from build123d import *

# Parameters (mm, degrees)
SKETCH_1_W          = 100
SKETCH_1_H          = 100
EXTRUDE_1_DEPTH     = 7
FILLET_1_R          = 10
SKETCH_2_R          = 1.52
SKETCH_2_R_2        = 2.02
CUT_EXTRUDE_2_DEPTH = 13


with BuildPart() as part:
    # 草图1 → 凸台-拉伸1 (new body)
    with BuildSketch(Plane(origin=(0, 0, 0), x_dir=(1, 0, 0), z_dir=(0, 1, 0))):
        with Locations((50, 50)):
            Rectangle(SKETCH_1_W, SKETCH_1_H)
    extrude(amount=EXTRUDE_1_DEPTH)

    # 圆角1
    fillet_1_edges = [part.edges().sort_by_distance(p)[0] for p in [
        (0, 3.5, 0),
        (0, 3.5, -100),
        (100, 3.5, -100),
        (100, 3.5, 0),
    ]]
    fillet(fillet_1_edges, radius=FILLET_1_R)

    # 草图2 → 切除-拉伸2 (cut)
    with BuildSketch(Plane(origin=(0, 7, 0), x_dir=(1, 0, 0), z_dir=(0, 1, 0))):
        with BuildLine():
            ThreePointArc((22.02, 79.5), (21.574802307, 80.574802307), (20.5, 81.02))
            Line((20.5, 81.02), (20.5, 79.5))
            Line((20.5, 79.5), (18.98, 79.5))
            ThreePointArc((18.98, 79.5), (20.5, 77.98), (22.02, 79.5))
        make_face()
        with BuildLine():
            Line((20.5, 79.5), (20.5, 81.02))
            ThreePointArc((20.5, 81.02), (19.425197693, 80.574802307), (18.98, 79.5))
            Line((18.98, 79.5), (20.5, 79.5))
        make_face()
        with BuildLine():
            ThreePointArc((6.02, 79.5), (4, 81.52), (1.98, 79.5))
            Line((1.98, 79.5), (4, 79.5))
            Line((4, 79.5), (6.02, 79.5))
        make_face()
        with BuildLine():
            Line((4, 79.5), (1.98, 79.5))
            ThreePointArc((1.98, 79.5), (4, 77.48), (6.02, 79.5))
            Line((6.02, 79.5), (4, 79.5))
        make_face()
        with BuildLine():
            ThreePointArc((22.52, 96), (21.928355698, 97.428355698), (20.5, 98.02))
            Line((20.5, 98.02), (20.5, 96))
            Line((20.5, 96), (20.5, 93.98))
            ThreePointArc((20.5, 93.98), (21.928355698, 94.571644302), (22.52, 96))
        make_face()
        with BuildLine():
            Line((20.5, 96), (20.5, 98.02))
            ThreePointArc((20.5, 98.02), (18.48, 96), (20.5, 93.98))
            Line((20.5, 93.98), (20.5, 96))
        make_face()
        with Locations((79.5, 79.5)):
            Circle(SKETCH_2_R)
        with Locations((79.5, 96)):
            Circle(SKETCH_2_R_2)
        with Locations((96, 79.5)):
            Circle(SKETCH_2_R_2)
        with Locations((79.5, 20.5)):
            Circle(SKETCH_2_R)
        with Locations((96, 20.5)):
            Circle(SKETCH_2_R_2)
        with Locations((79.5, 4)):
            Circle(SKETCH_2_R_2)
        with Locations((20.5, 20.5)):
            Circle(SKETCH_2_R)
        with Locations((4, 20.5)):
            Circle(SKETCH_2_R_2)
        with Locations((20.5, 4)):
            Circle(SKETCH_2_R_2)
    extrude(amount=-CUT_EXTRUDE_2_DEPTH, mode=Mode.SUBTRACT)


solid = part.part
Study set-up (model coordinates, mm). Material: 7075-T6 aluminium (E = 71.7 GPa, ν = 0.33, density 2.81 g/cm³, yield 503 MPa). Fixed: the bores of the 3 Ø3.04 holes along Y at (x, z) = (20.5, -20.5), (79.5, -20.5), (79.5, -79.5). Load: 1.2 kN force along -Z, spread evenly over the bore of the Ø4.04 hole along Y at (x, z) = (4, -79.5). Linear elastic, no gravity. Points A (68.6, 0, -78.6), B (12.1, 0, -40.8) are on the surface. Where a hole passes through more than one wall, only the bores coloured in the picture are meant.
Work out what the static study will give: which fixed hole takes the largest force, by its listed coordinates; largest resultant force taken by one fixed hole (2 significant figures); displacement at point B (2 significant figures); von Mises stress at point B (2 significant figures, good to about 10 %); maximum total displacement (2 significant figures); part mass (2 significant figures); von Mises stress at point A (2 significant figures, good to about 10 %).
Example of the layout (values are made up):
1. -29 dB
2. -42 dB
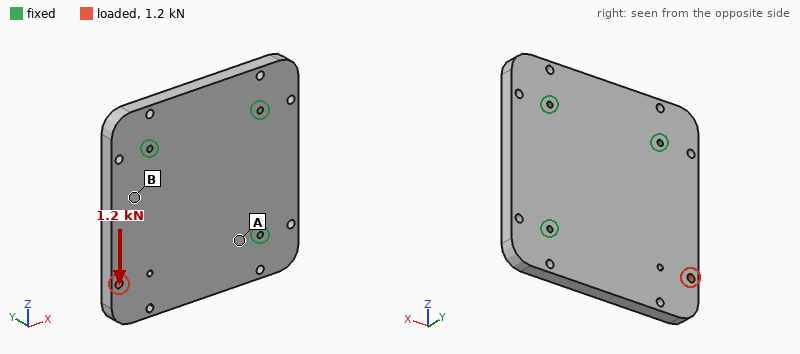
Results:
1. (20.5, -20.5)
2. 1.1 kN
3. 2.6 µm
4. 5.9 MPa
5. 8.9 µm
6. 190 g
7. 2.7 MPa
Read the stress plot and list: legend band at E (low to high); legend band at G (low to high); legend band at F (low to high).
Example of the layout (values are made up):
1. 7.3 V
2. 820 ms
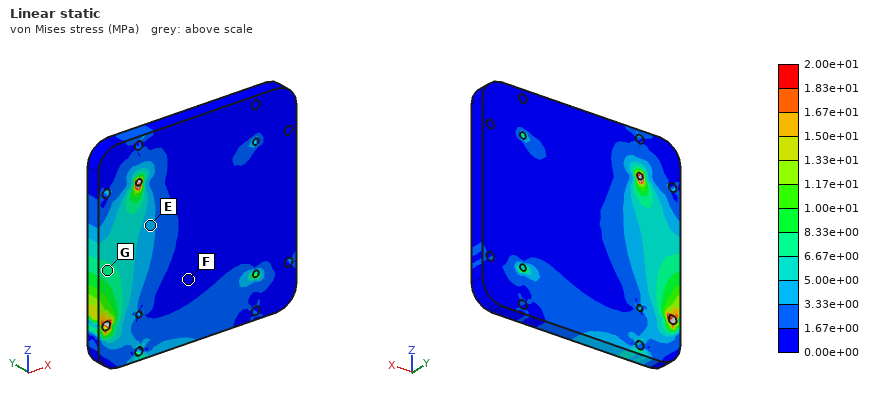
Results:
1. 3.33e+00 to 5.00e+00 MPa
2. 6.67e+00 to 8.33e+00 MPa
3. 0.00e+00 to 1.67e+00 MPa
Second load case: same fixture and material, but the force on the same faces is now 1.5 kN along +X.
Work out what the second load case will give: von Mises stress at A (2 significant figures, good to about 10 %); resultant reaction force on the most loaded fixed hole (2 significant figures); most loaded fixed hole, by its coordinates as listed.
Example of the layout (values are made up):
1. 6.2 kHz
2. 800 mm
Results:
1. 6.9 MPa
2. 1.1 kN
3. (79.5, -79.5)
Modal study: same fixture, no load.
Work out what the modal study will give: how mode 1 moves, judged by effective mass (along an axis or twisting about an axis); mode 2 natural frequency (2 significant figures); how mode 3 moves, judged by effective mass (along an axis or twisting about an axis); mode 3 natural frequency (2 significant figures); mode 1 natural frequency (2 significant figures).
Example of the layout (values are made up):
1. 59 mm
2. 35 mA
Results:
1. along Y
2. 4900 Hz
3. along Y
4. 5400 Hz
5. 1600 Hz
